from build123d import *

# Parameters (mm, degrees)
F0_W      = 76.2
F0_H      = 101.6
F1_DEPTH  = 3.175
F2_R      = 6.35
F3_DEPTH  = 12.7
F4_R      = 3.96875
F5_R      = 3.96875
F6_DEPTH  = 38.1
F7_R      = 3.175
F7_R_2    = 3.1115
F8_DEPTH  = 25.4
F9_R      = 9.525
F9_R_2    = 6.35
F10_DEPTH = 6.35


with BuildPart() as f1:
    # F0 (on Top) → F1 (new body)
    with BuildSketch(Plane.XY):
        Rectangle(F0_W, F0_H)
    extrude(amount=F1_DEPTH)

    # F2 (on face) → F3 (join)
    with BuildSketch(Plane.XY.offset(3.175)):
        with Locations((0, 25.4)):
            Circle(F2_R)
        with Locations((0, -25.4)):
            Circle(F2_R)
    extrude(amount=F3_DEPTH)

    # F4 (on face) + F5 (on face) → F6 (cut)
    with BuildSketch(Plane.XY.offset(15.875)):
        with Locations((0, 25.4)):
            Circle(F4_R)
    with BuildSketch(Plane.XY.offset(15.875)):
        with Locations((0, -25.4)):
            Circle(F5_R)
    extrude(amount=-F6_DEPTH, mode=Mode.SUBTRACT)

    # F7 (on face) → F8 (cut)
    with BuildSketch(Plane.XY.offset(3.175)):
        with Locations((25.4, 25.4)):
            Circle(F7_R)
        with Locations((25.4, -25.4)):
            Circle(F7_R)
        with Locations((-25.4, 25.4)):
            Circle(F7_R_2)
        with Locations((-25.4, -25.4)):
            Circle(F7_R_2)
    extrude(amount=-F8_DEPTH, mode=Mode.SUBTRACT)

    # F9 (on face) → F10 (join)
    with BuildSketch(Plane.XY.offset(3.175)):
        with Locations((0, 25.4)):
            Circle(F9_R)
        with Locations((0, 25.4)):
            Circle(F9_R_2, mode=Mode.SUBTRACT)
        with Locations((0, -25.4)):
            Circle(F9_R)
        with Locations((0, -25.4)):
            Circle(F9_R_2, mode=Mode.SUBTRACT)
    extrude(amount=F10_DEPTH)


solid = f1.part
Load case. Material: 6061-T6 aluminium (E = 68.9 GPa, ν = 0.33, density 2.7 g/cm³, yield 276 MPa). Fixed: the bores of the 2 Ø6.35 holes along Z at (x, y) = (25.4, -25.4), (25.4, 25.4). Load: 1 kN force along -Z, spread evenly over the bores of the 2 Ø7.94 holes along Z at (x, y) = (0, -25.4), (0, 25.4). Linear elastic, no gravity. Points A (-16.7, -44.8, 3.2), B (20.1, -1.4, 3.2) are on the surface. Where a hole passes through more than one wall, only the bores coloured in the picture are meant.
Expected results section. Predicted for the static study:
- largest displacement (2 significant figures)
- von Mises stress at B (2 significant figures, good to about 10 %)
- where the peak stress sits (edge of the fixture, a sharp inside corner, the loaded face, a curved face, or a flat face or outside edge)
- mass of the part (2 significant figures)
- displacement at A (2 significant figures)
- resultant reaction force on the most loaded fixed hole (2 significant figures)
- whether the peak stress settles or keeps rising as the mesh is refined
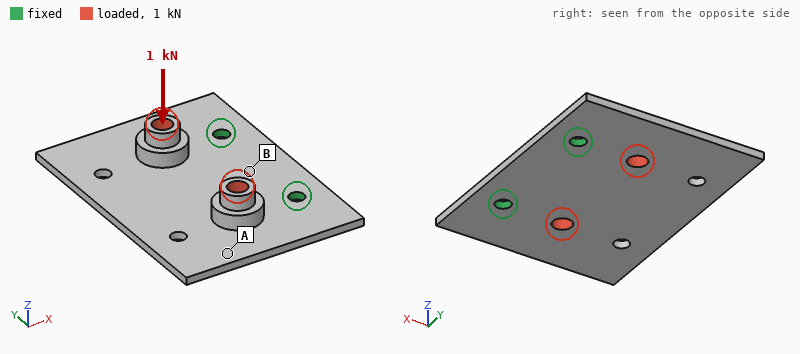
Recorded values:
1.1 mm
56 MPa
edge of the fixture
75 g
0.63 mm
500 N
keeps rising
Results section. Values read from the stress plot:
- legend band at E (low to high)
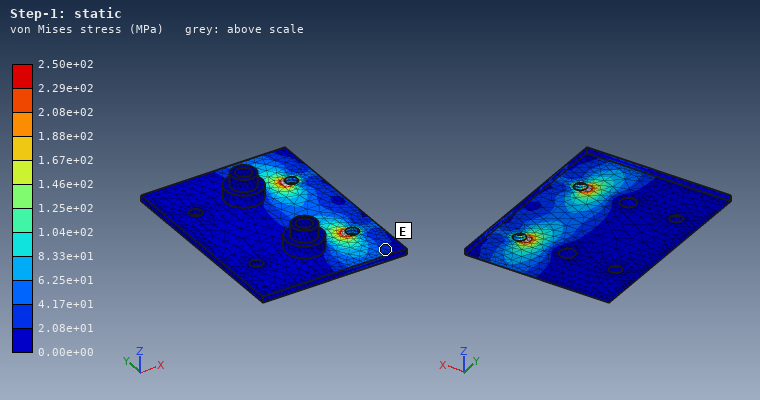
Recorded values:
2.08e+01 to 4.17e+01 MPa
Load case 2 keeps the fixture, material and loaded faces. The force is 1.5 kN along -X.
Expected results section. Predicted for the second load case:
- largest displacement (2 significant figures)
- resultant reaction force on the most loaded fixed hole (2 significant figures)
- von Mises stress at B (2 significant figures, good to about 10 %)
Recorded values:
0.61 mm
750 N
33 MPa
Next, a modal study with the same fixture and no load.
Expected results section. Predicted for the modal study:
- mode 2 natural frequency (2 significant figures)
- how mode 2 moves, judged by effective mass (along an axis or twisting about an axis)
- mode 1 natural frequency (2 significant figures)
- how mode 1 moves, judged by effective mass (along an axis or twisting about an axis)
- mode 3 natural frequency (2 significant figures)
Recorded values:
1100 Hz
twisting about X
640 Hz
along Z
2400 Hz
